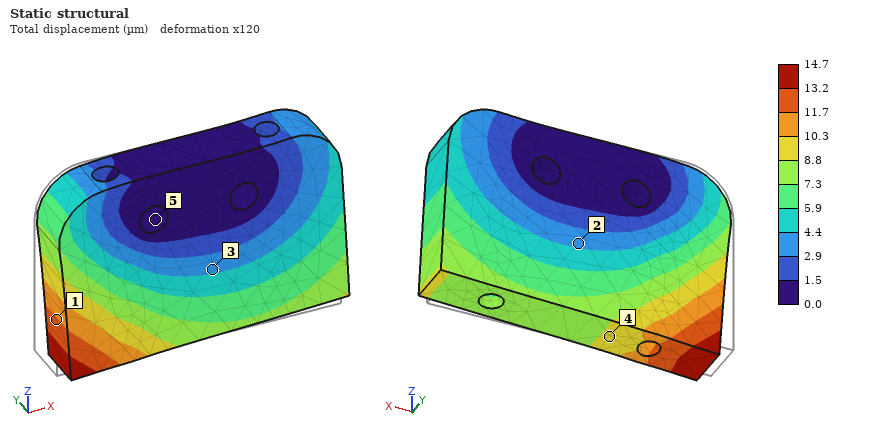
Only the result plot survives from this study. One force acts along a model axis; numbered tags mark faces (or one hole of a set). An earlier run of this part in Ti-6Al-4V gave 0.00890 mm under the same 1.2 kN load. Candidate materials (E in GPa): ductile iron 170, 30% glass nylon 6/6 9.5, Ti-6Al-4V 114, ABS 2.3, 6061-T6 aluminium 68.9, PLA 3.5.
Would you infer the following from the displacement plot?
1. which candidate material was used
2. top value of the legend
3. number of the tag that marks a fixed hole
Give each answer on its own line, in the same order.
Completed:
6061-T6 aluminium
14.7 µm
5
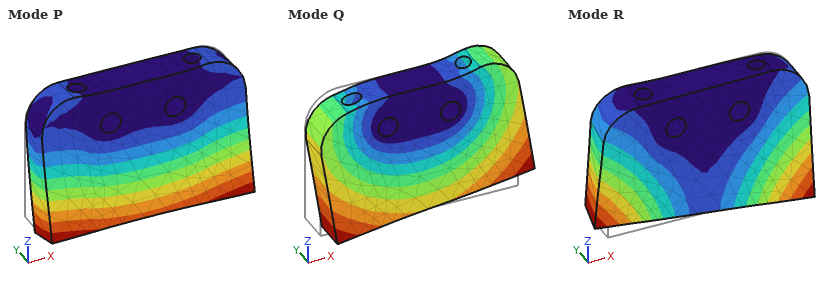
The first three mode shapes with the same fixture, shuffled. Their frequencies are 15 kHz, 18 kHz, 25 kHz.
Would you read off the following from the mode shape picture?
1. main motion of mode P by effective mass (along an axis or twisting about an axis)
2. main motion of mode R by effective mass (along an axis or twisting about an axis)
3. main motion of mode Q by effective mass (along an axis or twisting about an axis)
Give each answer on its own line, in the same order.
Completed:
along Y
twisting about Z
along X
